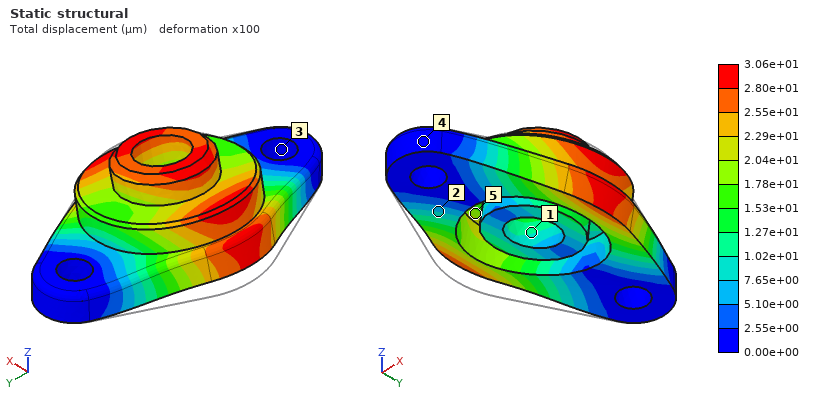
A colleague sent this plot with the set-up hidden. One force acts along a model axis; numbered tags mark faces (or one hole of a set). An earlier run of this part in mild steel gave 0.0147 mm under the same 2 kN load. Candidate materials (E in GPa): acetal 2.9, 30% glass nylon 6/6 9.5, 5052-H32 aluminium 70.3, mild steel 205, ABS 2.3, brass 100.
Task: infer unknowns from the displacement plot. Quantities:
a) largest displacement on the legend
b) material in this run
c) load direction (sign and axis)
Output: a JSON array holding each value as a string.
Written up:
["3.06e+01 µm", "brass", "+X"]
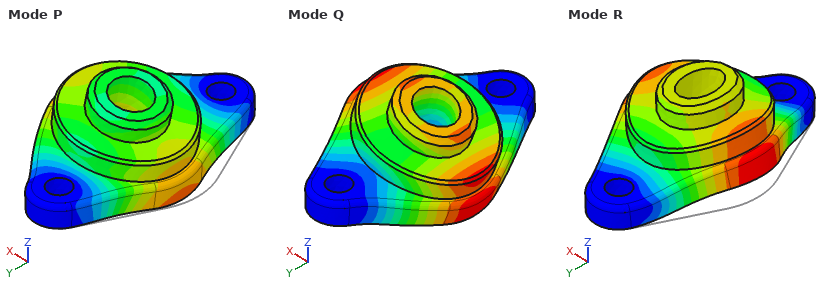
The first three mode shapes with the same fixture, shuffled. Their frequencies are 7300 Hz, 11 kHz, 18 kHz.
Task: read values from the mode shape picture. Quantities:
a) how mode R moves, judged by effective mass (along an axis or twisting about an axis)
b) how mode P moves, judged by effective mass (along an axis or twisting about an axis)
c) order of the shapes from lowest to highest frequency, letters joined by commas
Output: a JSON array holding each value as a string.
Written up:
["along Z", "along X", "Q, R, P"]
